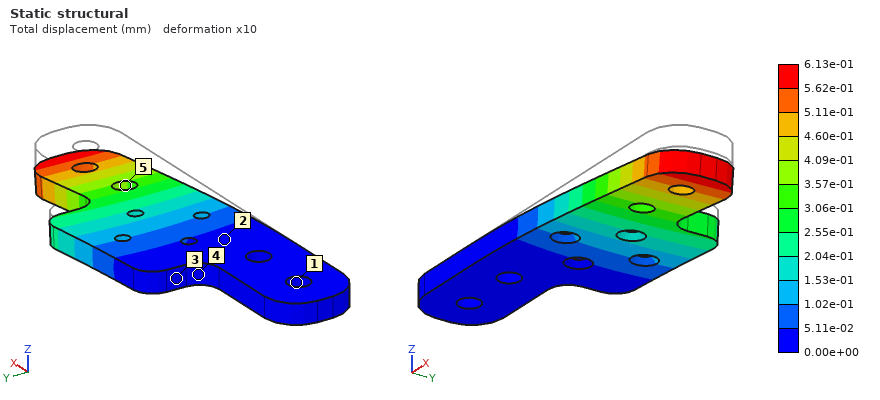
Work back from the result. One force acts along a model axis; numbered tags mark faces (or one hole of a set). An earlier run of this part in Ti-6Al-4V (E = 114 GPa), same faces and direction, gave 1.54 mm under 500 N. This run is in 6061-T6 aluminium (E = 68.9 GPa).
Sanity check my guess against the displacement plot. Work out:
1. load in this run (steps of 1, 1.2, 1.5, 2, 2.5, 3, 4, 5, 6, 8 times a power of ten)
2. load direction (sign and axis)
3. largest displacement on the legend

120 N
-Z
6.13e-01 mm
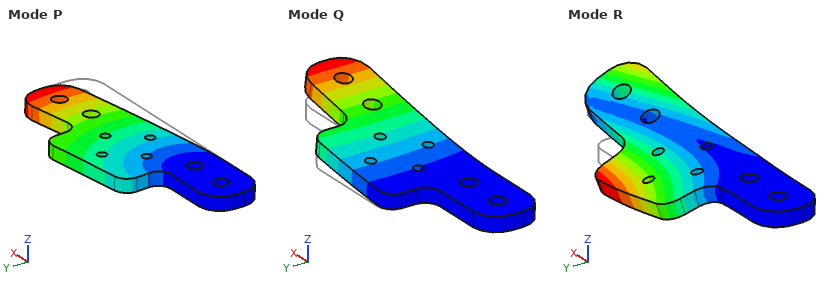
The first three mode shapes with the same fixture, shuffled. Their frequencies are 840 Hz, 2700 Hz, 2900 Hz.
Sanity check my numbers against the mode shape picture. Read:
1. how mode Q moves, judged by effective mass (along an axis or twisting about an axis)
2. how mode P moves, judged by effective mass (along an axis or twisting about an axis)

along Z
along Y
